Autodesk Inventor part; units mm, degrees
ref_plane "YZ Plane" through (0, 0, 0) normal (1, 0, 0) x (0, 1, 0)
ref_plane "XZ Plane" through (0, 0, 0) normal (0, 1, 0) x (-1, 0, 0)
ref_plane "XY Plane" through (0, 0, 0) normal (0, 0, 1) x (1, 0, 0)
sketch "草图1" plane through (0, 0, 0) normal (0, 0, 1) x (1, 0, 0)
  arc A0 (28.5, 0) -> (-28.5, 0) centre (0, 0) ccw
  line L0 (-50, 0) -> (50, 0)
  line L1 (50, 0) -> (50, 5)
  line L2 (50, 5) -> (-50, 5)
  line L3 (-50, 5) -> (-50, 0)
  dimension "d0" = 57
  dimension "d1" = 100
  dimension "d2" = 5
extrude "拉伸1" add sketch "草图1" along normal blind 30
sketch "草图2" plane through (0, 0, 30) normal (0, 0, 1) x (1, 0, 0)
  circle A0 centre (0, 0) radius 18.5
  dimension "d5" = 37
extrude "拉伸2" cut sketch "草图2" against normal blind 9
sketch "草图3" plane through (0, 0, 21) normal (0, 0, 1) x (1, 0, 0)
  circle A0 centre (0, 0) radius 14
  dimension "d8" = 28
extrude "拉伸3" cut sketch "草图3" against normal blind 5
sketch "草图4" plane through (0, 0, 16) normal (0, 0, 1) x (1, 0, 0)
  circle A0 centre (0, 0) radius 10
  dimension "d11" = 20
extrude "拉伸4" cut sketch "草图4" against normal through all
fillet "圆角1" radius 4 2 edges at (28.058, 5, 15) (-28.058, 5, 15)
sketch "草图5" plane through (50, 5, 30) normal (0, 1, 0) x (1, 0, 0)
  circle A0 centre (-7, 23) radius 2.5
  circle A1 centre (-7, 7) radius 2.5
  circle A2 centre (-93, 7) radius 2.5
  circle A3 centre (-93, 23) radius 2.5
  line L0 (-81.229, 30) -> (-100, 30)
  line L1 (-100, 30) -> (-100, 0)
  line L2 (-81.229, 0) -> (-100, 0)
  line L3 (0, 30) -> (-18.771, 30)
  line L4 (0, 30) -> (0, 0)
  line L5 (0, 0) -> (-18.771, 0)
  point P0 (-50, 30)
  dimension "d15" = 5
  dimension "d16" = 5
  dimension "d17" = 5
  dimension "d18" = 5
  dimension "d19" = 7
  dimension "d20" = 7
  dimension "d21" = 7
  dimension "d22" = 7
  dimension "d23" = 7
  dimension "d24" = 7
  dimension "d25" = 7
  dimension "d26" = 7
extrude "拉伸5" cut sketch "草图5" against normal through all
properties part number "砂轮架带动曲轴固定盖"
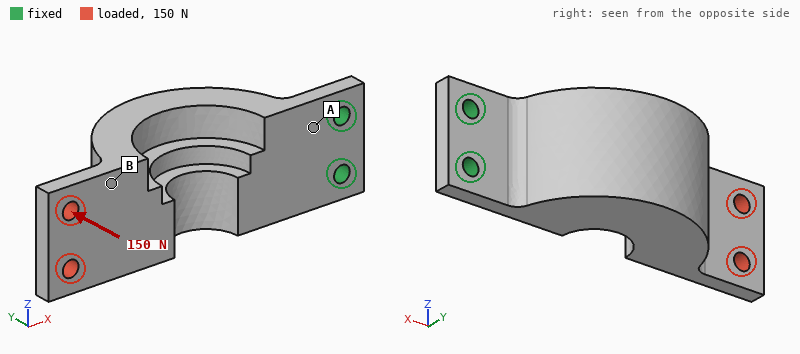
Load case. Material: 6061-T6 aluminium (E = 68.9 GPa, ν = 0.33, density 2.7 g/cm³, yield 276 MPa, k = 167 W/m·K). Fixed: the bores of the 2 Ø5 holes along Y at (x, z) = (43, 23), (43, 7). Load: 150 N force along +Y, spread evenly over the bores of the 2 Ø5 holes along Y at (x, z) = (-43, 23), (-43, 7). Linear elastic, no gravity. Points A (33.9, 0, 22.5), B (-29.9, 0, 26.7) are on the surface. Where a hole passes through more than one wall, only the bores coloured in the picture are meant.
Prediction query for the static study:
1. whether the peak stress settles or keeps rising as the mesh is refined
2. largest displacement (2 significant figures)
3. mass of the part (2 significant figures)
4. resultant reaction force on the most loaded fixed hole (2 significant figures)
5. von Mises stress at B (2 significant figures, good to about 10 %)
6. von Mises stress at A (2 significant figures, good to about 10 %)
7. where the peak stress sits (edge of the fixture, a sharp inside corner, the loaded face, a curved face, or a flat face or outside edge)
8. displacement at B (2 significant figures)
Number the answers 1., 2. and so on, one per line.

1. keeps rising
2. 0.71 mm
3. 96 g
4. 78 N
5. 12 MPa
6. 84 MPa
7. edge of the fixture
8. 0.53 mm
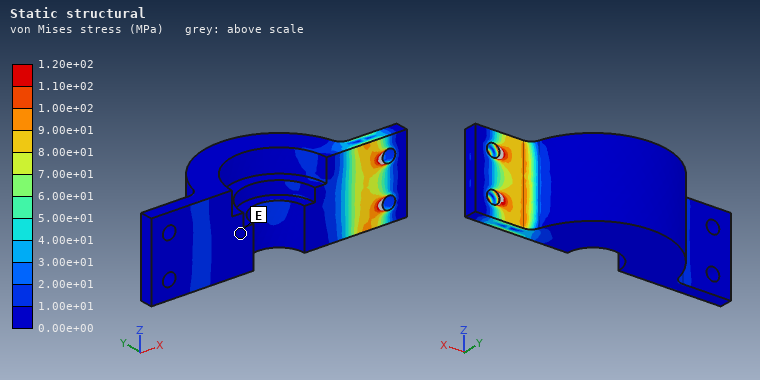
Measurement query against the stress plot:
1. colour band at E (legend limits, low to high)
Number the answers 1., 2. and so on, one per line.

1. 0.00e+00 to 1.00e+01 MPa
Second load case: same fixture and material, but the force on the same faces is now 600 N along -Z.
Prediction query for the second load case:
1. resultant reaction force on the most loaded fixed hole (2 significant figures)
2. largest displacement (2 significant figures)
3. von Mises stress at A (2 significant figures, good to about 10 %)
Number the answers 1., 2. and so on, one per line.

1. 2.7 kN
2. 0.24 mm
3. 38 MPa
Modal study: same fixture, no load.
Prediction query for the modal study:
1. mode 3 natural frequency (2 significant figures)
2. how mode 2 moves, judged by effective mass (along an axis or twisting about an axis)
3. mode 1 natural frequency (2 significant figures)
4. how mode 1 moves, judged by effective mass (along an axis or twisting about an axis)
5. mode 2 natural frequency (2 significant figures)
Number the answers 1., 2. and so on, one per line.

1. 2700 Hz
2. along Z
3. 460 Hz
4. along Y
5. 1800 Hz
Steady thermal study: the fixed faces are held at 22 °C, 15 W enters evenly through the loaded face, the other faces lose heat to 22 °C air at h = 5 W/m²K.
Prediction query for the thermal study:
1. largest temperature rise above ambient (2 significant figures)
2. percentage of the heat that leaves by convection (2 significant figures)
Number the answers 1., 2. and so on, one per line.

1. 34 K
2. 5.1 %
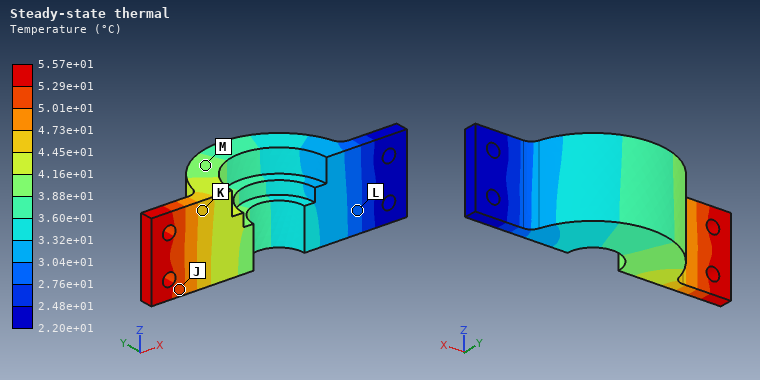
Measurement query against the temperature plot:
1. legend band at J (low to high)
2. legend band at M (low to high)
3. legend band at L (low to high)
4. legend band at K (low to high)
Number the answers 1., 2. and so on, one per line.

1. 5.01e+01 to 5.29e+01 °C
2. 3.88e+01 to 4.16e+01 °C
3. 2.76e+01 to 3.04e+01 °C
4. 4.45e+01 to 4.73e+01 °C
